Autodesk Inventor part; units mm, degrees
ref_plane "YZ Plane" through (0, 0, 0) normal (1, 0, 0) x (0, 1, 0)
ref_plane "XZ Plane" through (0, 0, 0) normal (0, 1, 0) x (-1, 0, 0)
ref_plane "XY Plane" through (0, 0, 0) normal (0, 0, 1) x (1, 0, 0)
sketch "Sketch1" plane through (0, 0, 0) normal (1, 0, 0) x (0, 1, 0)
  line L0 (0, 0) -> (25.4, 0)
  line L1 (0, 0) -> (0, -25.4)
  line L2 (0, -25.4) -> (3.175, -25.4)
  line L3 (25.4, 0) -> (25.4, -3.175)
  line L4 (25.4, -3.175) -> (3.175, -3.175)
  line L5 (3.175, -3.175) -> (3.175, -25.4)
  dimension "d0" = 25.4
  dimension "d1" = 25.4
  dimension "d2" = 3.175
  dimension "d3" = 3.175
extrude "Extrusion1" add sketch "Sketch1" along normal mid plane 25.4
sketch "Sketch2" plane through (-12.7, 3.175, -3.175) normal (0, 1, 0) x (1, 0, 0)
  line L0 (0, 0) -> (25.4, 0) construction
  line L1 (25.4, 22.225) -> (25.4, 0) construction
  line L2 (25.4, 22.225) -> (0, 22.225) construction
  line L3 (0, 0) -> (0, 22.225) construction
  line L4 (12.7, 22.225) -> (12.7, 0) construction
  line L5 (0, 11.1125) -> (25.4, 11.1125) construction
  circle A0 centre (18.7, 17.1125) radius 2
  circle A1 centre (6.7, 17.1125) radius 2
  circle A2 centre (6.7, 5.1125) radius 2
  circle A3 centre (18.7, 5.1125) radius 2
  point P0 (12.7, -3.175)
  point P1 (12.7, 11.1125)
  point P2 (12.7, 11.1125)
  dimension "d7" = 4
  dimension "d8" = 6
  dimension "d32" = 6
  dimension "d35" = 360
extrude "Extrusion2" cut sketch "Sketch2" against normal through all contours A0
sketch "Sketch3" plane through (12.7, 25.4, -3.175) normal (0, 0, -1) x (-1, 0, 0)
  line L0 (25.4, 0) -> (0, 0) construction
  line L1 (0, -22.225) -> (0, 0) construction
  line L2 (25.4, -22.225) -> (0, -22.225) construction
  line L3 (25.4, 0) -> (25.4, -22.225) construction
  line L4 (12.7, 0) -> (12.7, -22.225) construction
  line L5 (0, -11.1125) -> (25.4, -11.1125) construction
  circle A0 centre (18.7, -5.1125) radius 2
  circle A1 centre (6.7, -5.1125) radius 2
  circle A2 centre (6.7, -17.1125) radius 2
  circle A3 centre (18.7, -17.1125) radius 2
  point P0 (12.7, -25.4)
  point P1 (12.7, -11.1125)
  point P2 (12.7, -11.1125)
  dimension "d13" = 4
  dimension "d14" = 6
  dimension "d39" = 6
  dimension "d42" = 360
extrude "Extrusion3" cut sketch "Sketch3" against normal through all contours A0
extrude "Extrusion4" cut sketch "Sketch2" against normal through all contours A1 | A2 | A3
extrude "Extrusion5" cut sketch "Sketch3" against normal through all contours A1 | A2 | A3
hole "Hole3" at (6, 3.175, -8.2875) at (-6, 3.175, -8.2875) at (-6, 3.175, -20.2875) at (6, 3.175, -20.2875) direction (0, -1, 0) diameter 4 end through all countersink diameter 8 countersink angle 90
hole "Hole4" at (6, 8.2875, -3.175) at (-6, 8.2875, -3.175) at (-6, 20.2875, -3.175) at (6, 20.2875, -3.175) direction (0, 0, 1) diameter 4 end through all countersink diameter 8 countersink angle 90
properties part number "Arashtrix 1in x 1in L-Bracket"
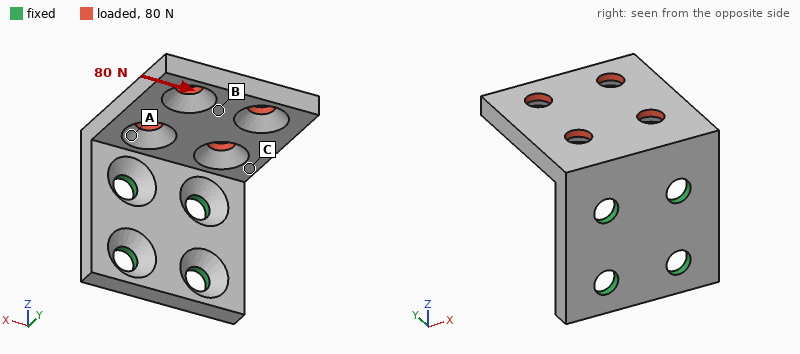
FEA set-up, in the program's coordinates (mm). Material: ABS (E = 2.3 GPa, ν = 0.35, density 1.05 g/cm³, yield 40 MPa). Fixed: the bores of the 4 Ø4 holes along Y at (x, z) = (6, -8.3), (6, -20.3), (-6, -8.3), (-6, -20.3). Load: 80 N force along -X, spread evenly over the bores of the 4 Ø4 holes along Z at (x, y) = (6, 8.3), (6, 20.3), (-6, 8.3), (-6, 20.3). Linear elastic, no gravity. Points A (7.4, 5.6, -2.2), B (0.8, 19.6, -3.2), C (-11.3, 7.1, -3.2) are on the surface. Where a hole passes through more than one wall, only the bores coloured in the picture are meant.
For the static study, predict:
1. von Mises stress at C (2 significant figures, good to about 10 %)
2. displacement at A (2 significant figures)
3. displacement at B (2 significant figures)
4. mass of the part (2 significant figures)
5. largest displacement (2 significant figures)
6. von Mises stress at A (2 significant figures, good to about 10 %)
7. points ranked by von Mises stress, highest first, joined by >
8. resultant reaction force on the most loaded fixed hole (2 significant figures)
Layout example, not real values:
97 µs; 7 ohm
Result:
7.5 MPa; 0.11 mm; 0.26 mm; 3.4 g; 0.38 mm; 4.0 MPa; C > A > B; 110 N
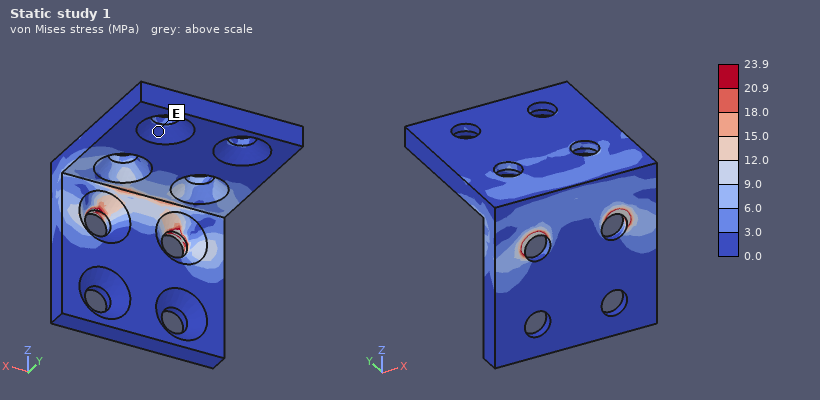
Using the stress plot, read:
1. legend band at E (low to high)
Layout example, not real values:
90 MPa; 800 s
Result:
0.0 to 3.0 MPa
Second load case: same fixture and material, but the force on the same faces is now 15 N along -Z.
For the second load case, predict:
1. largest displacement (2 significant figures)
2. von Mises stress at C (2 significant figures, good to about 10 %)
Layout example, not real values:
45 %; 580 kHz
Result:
0.48 mm; 4.0 MPa
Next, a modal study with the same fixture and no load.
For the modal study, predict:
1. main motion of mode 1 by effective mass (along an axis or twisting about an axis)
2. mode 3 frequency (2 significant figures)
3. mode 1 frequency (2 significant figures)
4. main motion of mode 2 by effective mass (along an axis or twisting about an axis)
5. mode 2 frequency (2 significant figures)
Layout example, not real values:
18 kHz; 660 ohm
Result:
along Z; 2800 Hz; 860 Hz; along X; 1900 Hz
